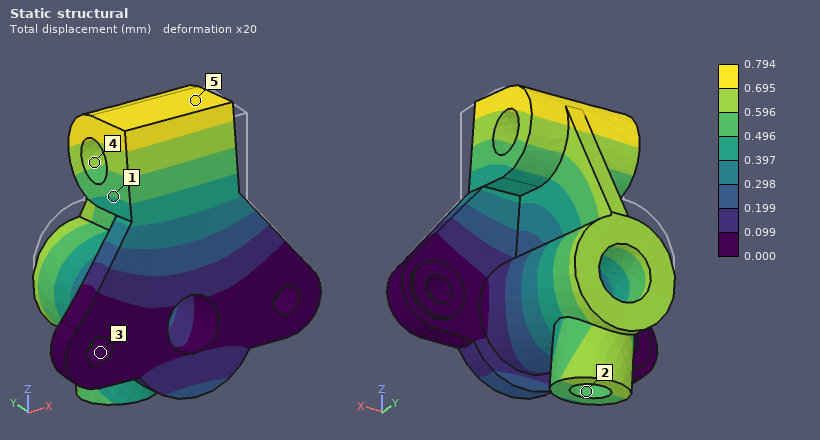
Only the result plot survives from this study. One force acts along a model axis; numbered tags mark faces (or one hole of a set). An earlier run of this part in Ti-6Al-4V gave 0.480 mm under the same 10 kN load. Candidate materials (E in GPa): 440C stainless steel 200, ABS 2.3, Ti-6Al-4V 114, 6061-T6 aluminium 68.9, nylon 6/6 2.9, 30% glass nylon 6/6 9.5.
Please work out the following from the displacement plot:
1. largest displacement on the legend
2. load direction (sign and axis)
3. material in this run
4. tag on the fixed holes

0.794 mm
+Y
6061-T6 aluminium
3
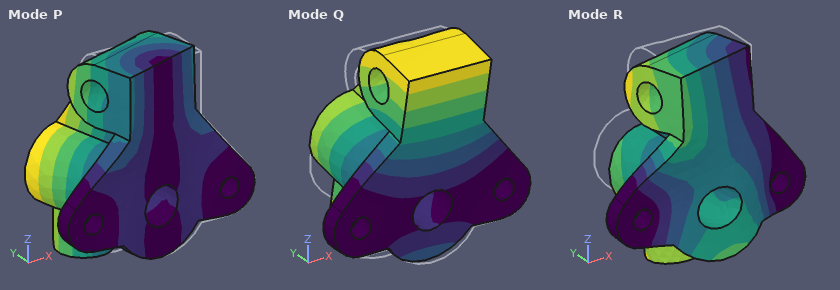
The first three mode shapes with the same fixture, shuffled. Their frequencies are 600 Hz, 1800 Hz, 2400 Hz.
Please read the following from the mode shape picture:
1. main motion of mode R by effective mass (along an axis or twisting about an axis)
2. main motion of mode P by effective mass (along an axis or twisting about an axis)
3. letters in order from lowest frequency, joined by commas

along Y
along X
Q, P, R
